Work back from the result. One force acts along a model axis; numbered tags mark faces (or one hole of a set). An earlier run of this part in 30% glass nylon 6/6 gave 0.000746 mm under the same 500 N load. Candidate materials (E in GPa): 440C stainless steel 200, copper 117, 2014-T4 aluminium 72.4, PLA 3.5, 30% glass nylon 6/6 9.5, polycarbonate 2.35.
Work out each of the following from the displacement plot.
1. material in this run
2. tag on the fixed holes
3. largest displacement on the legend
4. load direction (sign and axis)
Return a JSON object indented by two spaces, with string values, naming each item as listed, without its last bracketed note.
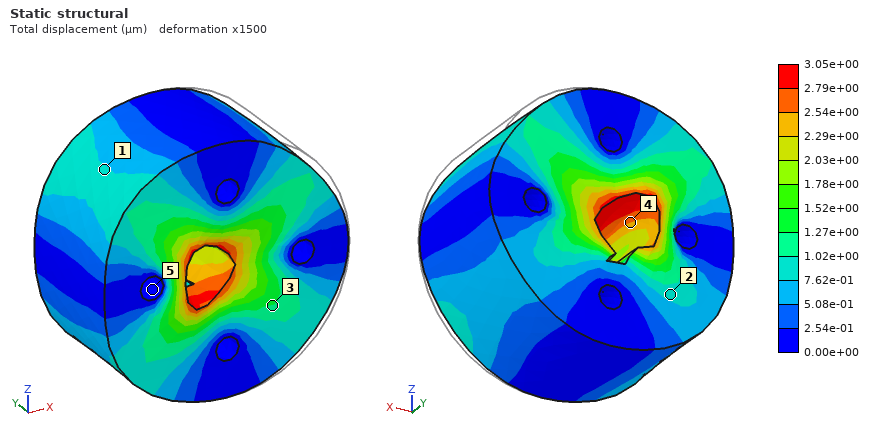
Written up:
{
  "material in this run": "polycarbonate",
  "tag on the fixed holes": "5",
  "largest displacement on the legend": "3.05e+00 µm",
  "load direction": "-X"
}
